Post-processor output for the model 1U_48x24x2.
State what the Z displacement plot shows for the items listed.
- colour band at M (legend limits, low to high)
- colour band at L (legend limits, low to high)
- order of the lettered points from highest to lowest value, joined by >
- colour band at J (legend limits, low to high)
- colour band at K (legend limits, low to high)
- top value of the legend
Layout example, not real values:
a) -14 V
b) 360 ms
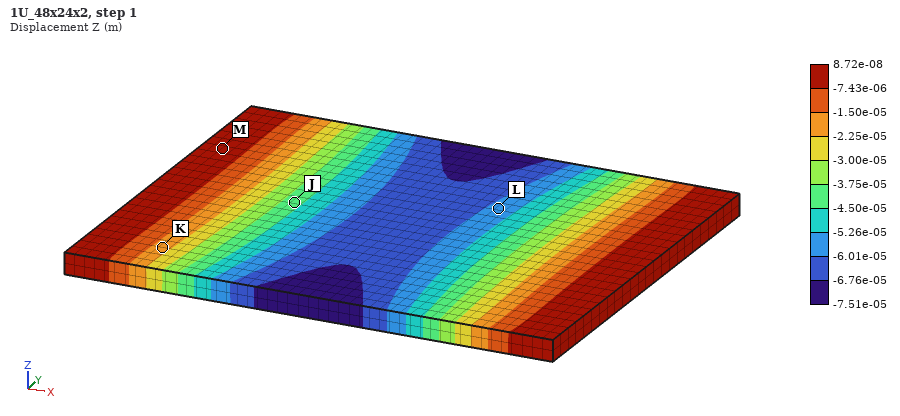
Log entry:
a) -7.43e-06 to 8.72e-08 m
b) -6.01e-05 to -5.26e-05 m
c) M > K > J > L
d) -4.50e-05 to -3.75e-05 m
e) -2.25e-05 to -1.50e-05 m
f) 8.72e-08 m
